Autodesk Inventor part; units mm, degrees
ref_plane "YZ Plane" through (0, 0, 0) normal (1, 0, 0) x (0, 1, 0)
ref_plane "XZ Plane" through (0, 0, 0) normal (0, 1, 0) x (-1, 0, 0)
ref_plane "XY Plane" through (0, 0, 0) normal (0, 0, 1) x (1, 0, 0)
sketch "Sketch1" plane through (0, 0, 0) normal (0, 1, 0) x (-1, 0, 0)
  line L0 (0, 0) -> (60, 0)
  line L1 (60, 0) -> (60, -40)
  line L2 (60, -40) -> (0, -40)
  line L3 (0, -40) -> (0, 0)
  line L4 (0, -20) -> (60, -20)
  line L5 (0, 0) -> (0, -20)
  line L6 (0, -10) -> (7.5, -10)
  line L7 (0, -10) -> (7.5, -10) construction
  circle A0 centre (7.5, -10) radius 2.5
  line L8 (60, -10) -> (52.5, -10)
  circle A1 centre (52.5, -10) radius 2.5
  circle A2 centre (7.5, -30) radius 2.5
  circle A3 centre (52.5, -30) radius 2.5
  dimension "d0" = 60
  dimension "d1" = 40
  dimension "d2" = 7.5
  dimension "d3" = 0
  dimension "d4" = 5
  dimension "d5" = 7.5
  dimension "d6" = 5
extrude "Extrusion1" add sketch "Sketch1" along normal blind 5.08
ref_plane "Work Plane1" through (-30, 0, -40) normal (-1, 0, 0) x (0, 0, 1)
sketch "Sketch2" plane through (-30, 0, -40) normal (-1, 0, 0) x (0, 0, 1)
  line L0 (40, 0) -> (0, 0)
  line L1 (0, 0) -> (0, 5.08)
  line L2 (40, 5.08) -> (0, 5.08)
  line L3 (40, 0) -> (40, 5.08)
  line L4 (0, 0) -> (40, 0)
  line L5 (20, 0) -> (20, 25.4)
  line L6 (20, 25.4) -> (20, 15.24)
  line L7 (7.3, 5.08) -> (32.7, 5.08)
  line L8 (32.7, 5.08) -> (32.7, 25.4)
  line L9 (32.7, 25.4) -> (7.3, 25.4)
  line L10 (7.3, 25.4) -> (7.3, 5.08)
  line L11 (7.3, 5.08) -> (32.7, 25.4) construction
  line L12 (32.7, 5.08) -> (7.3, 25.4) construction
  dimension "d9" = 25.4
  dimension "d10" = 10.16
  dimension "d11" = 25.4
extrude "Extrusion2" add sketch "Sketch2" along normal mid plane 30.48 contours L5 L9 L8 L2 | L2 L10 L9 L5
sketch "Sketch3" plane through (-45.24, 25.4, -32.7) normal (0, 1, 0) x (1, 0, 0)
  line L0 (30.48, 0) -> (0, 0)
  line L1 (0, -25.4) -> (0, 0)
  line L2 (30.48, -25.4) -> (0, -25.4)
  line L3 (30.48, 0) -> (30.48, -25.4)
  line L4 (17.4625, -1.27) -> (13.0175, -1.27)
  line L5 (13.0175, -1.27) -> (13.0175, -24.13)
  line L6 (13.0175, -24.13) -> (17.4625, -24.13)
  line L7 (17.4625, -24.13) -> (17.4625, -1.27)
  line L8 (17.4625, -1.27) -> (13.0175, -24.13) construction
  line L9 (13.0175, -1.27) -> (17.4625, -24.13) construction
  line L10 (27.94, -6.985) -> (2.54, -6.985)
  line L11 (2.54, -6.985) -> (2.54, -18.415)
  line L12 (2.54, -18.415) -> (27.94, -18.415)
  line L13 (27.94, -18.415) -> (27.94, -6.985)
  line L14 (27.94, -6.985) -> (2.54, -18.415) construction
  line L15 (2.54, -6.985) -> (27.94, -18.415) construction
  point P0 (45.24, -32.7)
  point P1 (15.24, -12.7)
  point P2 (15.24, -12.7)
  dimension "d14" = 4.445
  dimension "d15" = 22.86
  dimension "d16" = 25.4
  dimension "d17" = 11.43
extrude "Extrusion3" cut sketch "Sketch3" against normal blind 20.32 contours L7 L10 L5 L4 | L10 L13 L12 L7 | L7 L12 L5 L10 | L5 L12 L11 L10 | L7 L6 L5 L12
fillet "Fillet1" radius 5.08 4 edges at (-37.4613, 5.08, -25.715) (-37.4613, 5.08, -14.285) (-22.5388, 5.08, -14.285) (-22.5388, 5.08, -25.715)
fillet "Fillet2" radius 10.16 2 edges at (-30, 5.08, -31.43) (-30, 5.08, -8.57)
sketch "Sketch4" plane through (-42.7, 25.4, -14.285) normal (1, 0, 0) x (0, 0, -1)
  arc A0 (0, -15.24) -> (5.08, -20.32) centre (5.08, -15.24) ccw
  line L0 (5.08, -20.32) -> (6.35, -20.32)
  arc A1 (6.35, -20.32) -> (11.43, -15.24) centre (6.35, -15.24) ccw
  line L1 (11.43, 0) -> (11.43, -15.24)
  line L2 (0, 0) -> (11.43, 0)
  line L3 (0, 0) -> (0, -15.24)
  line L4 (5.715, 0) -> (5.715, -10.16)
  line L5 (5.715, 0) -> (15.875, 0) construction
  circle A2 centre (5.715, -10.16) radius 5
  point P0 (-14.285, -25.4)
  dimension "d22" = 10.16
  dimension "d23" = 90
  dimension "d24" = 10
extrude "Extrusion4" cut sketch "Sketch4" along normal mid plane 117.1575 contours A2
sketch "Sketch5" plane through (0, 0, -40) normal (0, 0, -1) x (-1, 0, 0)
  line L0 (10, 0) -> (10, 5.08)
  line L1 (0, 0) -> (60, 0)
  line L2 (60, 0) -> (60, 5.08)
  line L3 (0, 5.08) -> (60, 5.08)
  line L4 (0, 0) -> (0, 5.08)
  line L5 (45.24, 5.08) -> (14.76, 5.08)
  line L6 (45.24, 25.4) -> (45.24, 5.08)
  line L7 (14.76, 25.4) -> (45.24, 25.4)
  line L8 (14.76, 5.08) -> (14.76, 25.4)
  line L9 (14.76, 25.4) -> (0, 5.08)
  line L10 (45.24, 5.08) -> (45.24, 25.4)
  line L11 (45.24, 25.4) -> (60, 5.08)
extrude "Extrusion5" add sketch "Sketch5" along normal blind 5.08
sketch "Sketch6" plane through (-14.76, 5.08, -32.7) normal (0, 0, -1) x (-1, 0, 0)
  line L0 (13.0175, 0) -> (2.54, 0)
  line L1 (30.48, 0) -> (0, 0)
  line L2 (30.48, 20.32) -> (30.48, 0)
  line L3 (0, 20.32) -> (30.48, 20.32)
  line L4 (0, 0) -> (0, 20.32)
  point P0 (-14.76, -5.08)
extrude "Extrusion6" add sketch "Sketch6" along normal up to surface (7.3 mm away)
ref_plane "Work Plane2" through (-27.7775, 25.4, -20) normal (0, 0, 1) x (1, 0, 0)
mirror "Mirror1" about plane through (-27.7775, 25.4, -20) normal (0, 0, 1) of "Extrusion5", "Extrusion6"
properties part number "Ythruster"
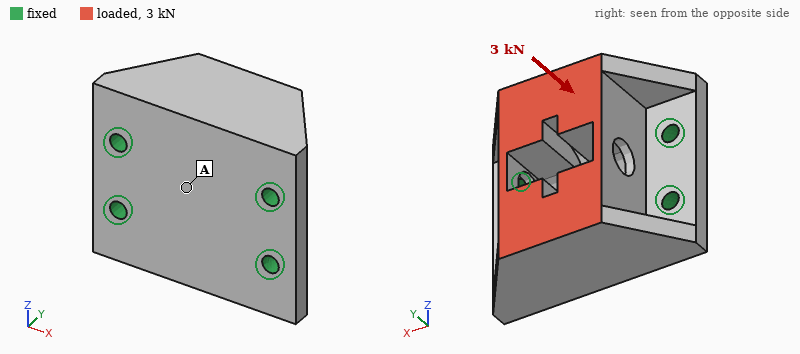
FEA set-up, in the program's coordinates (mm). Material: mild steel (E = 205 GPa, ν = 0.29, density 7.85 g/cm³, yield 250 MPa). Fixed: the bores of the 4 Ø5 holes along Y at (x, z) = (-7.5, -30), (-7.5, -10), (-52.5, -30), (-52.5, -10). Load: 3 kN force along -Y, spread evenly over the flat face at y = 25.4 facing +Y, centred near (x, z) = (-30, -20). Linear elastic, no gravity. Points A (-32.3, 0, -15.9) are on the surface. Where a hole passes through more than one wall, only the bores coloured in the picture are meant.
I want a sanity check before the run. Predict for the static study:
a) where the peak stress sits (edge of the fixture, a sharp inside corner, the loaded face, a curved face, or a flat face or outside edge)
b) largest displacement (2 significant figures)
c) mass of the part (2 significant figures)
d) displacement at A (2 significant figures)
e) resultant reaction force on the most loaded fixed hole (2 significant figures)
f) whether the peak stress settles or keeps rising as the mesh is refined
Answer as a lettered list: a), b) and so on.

a) edge of the fixture
b) 2.9 µm
c) 330 g
d) 2.1 µm
e) 810 N
f) keeps rising
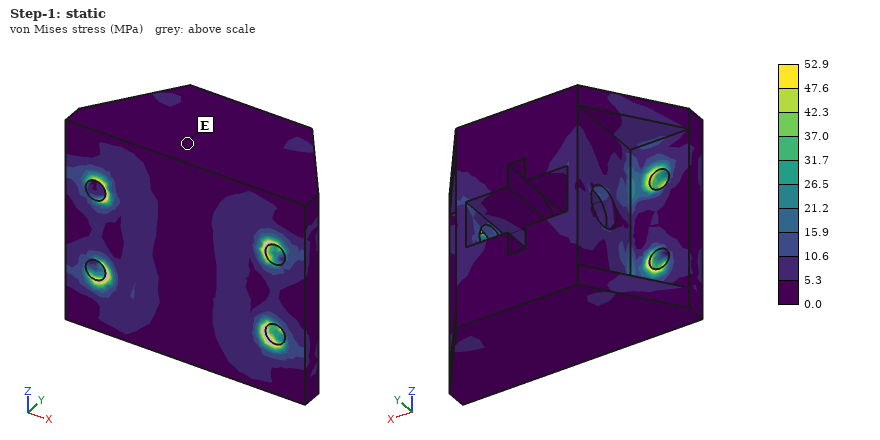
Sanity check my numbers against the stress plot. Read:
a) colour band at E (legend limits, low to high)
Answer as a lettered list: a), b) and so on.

a) 0.0 to 5.3 MPa
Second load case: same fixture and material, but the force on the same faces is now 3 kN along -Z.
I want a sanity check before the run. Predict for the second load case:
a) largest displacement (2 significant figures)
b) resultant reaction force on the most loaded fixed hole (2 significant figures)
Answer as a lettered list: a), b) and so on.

a) 16 µm
b) 1.5 kN
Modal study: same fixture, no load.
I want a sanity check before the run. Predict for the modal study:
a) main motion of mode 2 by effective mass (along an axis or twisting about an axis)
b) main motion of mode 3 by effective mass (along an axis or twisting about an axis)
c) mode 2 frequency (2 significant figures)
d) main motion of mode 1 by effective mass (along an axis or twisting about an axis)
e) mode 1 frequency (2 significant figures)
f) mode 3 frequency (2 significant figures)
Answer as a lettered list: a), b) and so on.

a) along Y
b) along X
c) 11 kHz
d) along Z
e) 6400 Hz
f) 13 kHz
